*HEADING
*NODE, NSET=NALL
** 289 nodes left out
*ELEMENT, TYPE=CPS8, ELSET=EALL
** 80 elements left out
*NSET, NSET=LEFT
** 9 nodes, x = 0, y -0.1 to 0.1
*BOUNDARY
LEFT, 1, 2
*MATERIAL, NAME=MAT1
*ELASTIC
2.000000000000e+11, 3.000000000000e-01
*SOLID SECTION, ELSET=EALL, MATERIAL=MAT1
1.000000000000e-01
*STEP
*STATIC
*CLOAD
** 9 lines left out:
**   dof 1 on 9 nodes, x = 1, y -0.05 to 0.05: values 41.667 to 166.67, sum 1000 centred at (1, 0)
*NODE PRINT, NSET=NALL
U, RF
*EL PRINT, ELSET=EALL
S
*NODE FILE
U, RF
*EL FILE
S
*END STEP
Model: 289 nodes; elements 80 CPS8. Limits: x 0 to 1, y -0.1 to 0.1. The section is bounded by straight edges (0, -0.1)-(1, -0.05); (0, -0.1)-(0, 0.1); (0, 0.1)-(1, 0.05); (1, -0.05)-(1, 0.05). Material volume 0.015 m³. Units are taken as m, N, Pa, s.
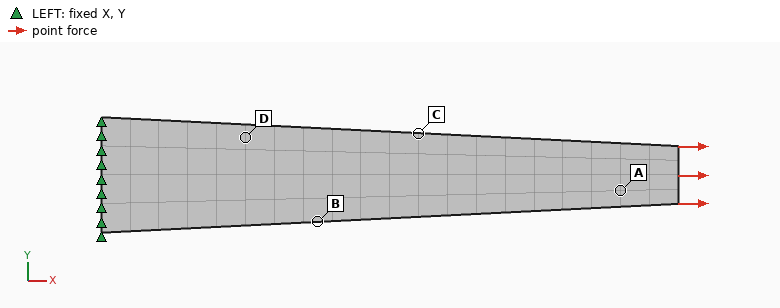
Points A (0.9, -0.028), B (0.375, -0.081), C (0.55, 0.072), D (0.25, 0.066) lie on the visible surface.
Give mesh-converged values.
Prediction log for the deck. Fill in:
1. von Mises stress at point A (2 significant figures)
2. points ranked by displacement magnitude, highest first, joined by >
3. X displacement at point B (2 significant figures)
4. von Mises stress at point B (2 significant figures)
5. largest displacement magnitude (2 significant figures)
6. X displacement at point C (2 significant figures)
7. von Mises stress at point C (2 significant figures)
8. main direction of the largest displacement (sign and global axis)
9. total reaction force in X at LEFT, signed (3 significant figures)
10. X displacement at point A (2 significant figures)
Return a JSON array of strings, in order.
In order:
["91000 Pa", "A > C > B > D", "1.0e-07 m", "61000 Pa", "3.5e-07 m", "1.6e-07 m", "69000 Pa", "+X", "-1000 N", "3.0e-07 m"]
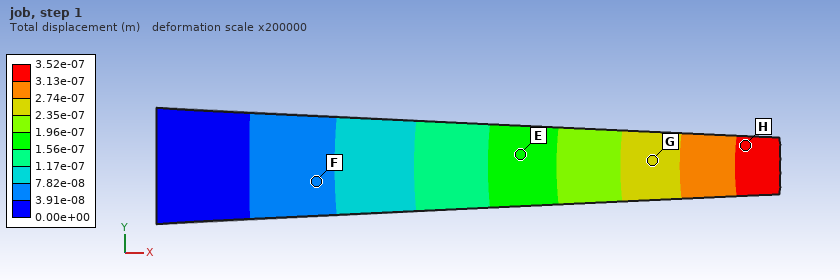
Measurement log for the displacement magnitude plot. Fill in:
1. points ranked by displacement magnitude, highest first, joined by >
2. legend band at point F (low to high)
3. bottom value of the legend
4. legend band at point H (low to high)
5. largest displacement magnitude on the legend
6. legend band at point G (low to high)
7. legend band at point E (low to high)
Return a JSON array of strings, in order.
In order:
["H > G > E > F", "3.91e-08 to 7.82e-08 m", "0.00e+00 m", "3.13e-07 to 3.52e-07 m", "3.52e-07 m", "2.35e-07 to 2.74e-07 m", "1.56e-07 to 1.96e-07 m"]
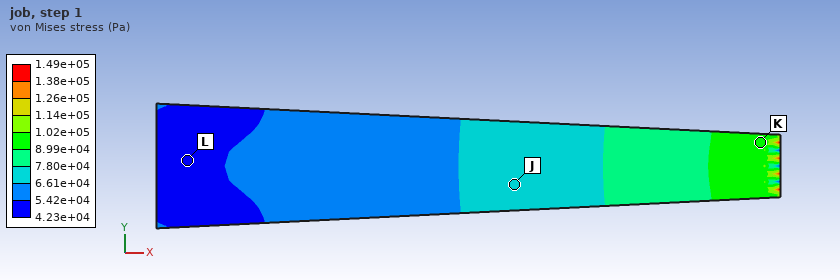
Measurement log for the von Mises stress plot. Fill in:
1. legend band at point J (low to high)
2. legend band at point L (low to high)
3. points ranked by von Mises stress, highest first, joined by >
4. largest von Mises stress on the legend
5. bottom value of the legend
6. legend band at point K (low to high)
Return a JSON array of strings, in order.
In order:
["6.61e+04 to 7.80e+04 Pa", "4.23e+04 to 5.42e+04 Pa", "K > J > L", "1.49e+05 Pa", "4.23e+04 Pa", "8.99e+04 to 1.02e+05 Pa"]
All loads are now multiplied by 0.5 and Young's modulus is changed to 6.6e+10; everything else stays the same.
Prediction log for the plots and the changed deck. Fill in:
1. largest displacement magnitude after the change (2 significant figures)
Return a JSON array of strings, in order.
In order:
["5.3e-07 m"]
